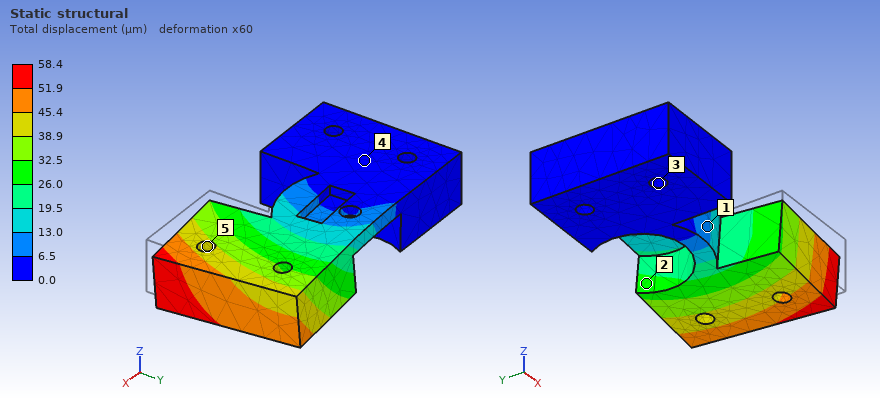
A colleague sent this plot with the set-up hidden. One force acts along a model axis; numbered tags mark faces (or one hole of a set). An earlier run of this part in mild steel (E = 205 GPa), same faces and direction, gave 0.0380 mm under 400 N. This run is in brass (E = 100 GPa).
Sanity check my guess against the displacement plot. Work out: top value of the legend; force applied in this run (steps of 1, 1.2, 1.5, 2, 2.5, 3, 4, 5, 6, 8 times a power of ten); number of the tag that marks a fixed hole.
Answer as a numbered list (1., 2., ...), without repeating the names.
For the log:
1. 58.4 µm
2. 300 N
3. 3
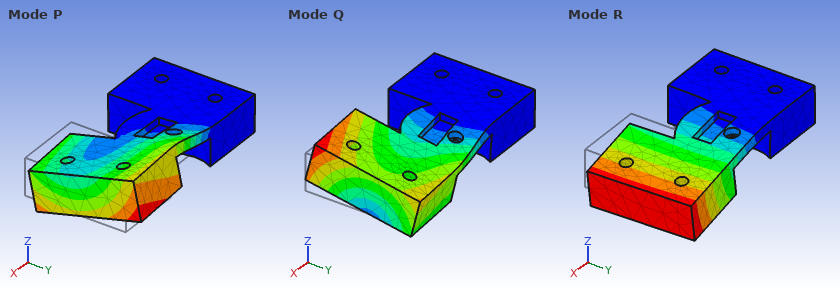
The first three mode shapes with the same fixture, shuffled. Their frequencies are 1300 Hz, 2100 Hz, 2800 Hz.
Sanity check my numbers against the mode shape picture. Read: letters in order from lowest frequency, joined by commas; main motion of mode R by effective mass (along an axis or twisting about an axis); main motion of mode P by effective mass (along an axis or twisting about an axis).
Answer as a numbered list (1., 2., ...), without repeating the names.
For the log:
1. R, P, Q
2. along Z
3. along Y
